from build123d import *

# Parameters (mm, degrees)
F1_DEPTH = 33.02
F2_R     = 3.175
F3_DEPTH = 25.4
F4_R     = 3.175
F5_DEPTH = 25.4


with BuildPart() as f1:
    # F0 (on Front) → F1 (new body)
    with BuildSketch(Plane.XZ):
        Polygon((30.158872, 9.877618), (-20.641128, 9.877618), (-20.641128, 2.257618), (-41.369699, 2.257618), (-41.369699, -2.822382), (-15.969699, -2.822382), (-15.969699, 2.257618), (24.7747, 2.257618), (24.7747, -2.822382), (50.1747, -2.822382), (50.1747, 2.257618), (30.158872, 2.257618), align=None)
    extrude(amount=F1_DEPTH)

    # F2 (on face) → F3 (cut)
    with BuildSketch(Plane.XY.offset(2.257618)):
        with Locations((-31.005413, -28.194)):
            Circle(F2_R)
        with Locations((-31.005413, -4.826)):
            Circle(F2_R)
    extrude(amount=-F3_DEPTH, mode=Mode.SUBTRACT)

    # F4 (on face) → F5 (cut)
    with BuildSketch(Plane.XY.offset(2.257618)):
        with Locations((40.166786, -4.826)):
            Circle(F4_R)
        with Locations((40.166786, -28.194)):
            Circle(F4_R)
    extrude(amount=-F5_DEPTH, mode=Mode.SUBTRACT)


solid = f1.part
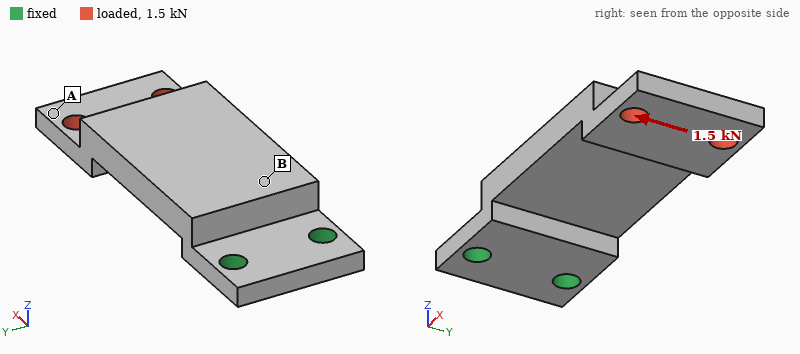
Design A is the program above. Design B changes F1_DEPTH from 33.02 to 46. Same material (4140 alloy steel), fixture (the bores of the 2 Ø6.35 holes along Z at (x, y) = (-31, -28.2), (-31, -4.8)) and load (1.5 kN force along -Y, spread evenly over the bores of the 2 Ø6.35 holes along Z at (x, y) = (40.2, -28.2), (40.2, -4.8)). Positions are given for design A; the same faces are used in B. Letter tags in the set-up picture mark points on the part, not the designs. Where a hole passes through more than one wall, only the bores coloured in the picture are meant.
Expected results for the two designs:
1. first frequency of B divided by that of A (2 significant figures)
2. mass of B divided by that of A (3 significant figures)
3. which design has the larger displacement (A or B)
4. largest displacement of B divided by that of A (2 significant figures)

0.97
1.41
A
0.67
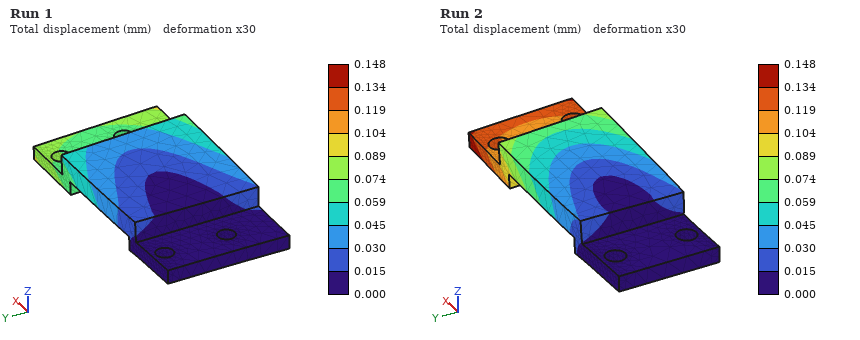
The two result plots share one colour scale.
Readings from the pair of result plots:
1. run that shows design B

Run 1
